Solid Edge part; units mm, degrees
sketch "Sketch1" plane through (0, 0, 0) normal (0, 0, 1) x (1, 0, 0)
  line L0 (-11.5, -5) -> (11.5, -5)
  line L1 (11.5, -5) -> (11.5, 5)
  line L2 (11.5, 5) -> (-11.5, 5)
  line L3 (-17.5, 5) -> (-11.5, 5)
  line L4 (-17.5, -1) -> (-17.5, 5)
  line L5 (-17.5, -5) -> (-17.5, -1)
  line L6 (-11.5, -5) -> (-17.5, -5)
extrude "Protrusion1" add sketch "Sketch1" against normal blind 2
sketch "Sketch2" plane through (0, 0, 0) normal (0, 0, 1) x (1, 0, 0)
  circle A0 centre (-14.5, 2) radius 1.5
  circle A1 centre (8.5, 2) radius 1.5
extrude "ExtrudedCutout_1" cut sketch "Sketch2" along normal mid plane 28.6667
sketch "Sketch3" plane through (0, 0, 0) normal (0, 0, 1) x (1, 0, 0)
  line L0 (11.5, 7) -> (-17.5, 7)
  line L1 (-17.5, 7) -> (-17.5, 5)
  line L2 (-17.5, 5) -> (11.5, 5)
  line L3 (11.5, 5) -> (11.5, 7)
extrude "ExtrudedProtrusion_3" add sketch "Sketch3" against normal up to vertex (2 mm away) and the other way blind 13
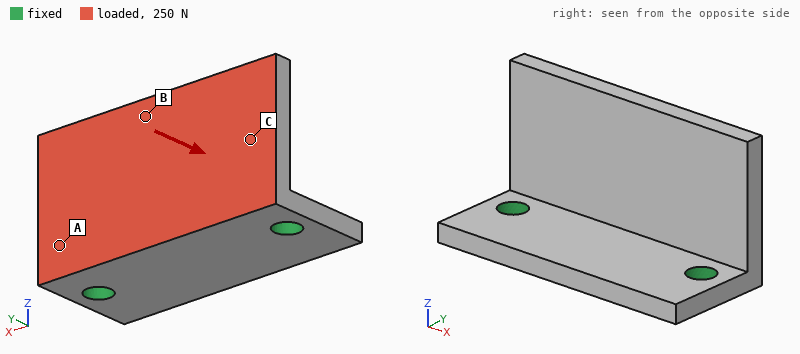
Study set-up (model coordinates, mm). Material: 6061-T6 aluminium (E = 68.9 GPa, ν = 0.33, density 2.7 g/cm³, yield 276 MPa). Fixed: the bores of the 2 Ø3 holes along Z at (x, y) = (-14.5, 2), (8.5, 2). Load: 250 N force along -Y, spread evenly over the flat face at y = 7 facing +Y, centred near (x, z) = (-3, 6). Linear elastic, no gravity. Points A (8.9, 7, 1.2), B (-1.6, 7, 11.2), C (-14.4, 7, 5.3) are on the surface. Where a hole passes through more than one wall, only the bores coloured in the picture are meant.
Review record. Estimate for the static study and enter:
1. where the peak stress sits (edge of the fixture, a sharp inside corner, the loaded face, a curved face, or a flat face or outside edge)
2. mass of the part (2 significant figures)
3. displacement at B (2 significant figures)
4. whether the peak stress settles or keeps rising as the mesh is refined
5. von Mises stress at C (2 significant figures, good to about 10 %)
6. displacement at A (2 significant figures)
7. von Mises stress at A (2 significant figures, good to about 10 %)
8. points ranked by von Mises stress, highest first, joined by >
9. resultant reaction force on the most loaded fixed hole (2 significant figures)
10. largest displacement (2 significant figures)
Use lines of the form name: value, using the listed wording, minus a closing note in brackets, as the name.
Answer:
where the peak stress sits: edge of the fixture
mass of the part: 3.8 g
displacement at B: 0.10 mm
whether the peak stress settles or keeps rising as the mesh is refined: keeps rising
von Mises stress at C: 28 MPa
displacement at A: 0.019 mm
von Mises stress at A: 62 MPa
points ranked by von Mises stress, highest first, joined by >: A > C > B
resultant reaction force on the most loaded fixed hole: 130 N
largest displacement: 0.12 mm
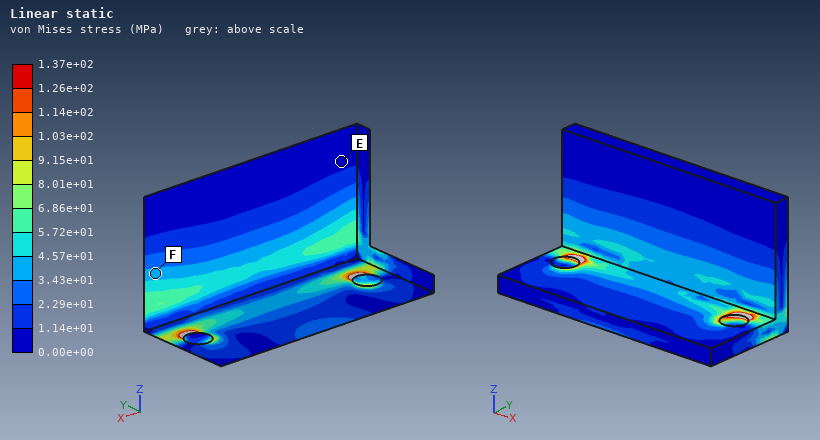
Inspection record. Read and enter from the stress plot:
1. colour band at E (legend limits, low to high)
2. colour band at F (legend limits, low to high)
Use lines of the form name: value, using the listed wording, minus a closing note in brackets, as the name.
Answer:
colour band at E: 0.00e+00 to 1.14e+01 MPa
colour band at F: 3.43e+01 to 4.57e+01 MPa
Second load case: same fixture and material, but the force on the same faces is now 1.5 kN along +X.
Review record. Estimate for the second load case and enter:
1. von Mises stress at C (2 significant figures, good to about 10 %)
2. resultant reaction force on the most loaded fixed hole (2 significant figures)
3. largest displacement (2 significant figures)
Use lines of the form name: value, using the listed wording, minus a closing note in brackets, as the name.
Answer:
von Mises stress at C: 26 MPa
resultant reaction force on the most loaded fixed hole: 900 N
largest displacement: 30 µm
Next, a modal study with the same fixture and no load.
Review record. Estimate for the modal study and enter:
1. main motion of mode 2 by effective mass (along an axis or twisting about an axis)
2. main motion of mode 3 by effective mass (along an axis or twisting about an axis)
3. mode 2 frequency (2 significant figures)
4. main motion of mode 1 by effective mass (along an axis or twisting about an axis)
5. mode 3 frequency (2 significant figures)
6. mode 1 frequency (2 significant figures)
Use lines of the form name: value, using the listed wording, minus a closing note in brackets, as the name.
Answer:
main motion of mode 2 by effective mass: twisting about Z
main motion of mode 3 by effective mass: along Z
mode 2 frequency: 10 kHz
main motion of mode 1 by effective mass: along Y
mode 3 frequency: 20 kHz
mode 1 frequency: 5900 Hz
